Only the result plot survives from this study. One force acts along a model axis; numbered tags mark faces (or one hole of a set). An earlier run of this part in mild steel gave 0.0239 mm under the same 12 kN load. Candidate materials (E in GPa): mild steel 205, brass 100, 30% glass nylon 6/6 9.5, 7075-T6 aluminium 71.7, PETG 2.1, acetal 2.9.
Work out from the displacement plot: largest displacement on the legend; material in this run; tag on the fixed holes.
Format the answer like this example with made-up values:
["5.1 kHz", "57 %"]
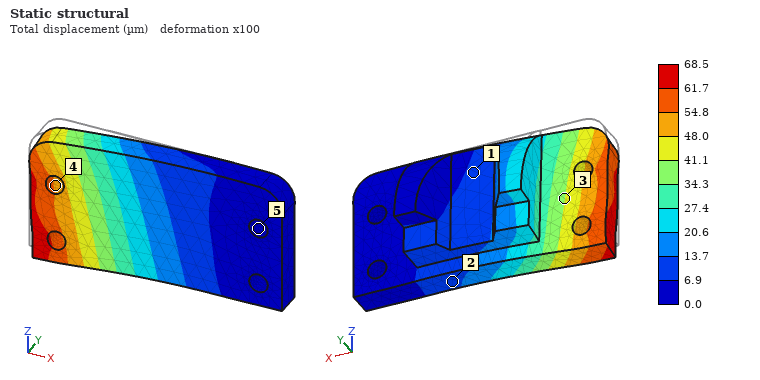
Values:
["68.5 µm", "7075-T6 aluminium", "5"]
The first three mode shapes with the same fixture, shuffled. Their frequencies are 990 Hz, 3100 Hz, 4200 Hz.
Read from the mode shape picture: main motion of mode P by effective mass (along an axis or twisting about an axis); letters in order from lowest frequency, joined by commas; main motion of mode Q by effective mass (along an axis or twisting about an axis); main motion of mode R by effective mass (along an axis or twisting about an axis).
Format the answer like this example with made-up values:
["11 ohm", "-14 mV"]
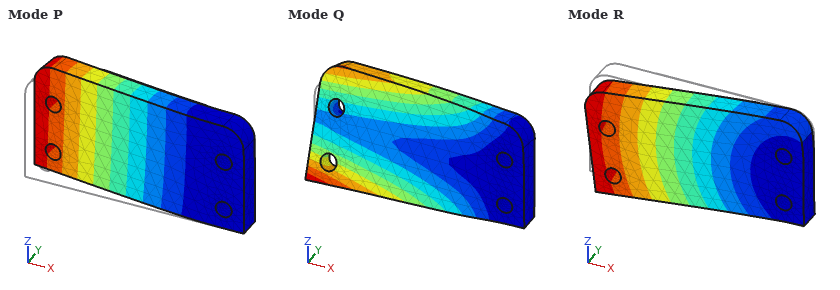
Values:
["along Y", "P, R, Q", "twisting about X", "along Z"]
